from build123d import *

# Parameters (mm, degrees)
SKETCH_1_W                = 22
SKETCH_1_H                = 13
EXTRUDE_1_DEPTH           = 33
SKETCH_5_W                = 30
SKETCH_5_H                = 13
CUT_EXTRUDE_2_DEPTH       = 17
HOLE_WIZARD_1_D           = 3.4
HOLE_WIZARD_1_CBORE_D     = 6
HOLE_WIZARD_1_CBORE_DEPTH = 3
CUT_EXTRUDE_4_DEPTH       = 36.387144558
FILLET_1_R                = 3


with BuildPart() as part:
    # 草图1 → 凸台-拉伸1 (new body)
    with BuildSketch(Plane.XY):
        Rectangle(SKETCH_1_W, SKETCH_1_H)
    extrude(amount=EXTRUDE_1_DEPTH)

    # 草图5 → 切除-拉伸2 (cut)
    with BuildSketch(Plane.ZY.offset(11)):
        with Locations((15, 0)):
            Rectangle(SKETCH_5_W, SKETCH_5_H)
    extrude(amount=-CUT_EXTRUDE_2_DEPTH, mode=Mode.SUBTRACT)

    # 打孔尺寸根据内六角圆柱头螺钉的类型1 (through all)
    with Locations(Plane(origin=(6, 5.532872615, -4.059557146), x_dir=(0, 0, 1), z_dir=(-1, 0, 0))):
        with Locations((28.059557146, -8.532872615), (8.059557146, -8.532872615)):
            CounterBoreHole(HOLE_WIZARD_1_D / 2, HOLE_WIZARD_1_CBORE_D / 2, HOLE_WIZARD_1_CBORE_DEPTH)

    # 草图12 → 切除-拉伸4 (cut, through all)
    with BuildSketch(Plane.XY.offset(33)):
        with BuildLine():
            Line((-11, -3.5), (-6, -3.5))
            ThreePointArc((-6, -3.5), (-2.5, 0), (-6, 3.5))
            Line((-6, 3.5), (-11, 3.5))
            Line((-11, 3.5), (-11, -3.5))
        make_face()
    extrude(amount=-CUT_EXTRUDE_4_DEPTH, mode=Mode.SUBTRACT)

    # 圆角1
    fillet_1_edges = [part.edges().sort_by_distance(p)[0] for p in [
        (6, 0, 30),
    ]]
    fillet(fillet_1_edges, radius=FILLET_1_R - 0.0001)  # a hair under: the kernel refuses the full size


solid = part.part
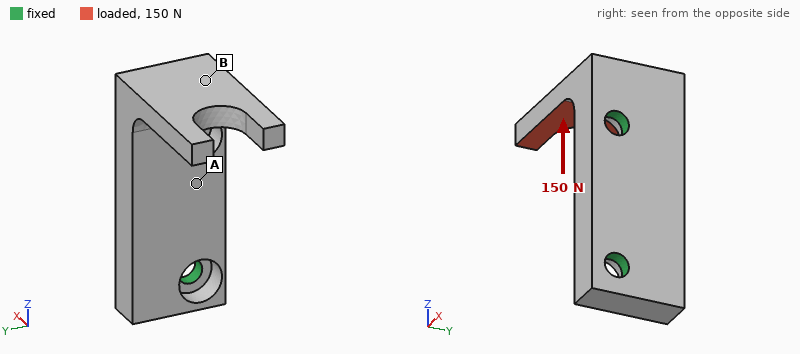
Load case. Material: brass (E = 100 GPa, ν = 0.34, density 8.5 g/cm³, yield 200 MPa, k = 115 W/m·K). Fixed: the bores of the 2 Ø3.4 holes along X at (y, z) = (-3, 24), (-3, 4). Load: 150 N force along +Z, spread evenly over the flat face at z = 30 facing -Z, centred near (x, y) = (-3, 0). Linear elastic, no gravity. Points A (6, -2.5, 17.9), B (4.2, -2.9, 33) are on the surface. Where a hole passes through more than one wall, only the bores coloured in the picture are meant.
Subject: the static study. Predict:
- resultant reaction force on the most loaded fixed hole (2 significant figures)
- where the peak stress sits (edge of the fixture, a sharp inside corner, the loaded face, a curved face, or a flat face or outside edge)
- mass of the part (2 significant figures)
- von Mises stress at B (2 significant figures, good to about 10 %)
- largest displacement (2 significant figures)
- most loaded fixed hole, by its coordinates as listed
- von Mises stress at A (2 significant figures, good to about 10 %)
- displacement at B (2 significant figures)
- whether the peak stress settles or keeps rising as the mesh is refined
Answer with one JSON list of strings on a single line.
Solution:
["160 N", "edge of the fixture", "21 g", "40 MPa", "65 µm", "(-3, 4)", "11 MPa", "15 µm", "keeps rising"]
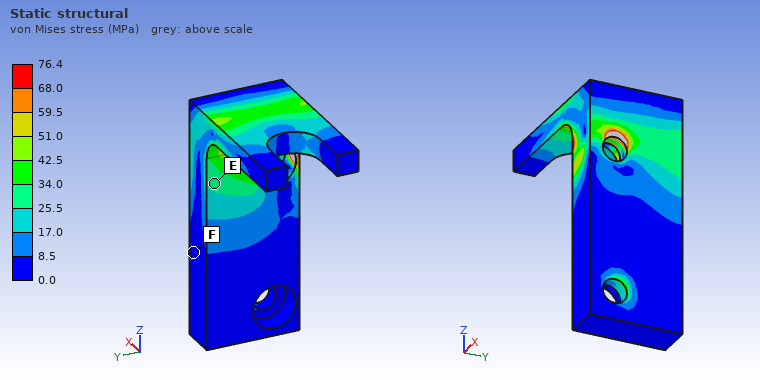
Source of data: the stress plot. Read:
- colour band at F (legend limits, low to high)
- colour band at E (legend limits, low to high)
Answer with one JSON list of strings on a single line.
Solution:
["0.0 to 8.5 MPa", "25.5 to 34.0 MPa"]
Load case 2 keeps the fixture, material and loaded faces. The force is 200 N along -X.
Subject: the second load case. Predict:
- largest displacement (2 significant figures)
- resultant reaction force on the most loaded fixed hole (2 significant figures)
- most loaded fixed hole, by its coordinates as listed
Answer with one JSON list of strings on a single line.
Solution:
["15 µm", "240 N", "(-3, 24)"]
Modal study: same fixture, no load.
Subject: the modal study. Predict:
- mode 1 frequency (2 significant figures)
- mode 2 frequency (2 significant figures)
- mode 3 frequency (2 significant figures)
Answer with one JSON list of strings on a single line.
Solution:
["4900 Hz", "5600 Hz", "10 kHz"]
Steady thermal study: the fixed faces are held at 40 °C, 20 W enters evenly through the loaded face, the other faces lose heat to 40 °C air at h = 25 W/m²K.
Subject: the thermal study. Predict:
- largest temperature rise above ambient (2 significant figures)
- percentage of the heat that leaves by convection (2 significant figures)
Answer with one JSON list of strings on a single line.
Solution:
["76 K", "4.1 %"]
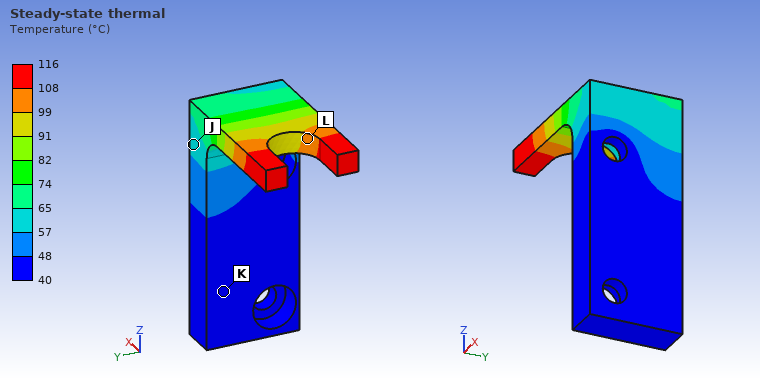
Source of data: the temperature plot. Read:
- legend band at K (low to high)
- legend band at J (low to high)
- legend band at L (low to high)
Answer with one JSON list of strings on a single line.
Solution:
["40 to 48 °C", "57 to 65 °C", "99 to 108 °C"]
